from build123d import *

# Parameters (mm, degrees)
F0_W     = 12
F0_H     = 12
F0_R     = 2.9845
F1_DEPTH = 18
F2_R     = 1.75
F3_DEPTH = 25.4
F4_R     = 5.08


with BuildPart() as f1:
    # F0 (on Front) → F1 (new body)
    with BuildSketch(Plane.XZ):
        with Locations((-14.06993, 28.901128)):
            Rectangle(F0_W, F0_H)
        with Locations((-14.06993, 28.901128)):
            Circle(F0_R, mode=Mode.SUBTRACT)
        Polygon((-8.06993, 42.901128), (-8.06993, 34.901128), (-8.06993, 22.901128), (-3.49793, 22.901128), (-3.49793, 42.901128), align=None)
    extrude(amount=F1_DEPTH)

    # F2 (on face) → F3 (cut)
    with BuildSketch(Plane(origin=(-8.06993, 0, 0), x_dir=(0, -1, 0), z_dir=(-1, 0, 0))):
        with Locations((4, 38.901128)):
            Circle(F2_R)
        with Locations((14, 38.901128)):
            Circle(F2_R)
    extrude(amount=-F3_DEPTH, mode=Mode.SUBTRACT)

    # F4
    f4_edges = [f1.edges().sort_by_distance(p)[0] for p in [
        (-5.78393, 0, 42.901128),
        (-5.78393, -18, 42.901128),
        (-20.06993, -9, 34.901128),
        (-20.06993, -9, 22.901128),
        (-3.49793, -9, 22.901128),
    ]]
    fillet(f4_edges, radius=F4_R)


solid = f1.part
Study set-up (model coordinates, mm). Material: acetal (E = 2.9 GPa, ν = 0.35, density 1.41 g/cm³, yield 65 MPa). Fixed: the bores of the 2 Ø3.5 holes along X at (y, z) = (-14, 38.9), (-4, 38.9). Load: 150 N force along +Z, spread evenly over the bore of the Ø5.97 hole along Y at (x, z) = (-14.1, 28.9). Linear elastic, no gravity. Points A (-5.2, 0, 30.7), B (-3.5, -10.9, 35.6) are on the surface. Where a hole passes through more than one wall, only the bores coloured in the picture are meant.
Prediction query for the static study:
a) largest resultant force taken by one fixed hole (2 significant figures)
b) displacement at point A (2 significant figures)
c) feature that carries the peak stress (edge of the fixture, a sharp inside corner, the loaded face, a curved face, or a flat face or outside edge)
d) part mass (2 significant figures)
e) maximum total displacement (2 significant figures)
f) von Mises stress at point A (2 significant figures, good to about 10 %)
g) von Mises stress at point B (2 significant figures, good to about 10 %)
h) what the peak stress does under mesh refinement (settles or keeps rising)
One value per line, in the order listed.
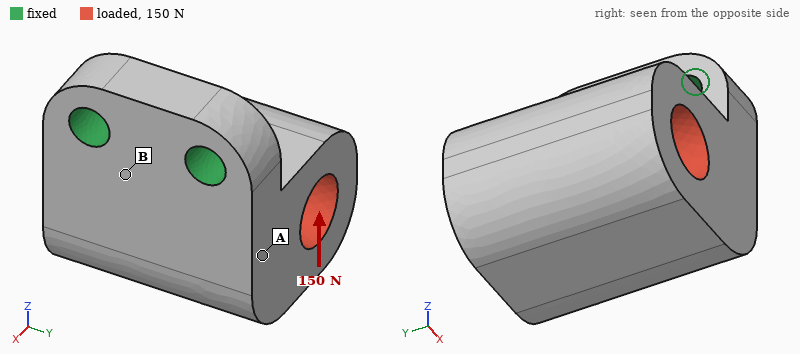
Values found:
76 N
0.073 mm
edge of the fixture
4.6 g
0.28 mm
4.2 MPa
14 MPa
keeps rising
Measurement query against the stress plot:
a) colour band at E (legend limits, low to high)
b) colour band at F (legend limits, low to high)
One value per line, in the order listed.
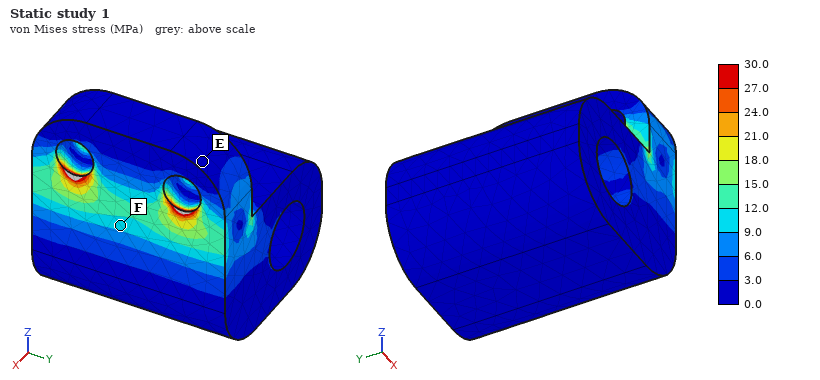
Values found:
0.0 to 3.0 MPa
9.0 to 12.0 MPa
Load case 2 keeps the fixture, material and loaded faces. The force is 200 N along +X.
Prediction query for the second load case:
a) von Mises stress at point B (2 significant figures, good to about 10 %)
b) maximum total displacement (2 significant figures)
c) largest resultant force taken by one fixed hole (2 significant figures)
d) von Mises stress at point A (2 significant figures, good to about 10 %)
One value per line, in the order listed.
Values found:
15 MPa
0.31 mm
100 N
4.4 MPa
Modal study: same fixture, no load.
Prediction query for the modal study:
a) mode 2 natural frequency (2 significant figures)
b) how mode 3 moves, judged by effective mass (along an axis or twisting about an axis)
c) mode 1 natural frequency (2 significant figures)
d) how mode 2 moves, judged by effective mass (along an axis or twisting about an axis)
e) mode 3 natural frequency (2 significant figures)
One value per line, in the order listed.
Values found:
4500 Hz
along Y
2100 Hz
along Y
7300 Hz
